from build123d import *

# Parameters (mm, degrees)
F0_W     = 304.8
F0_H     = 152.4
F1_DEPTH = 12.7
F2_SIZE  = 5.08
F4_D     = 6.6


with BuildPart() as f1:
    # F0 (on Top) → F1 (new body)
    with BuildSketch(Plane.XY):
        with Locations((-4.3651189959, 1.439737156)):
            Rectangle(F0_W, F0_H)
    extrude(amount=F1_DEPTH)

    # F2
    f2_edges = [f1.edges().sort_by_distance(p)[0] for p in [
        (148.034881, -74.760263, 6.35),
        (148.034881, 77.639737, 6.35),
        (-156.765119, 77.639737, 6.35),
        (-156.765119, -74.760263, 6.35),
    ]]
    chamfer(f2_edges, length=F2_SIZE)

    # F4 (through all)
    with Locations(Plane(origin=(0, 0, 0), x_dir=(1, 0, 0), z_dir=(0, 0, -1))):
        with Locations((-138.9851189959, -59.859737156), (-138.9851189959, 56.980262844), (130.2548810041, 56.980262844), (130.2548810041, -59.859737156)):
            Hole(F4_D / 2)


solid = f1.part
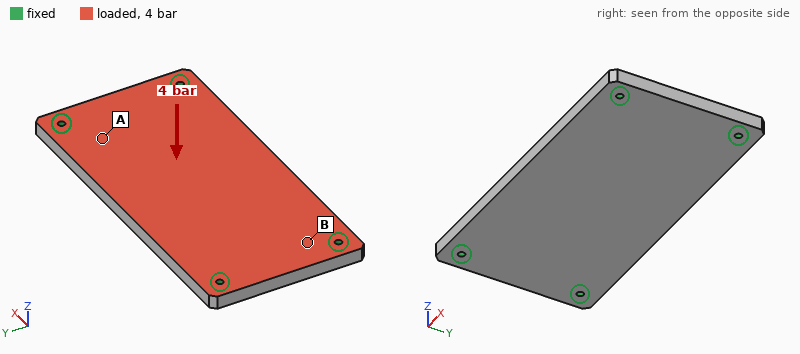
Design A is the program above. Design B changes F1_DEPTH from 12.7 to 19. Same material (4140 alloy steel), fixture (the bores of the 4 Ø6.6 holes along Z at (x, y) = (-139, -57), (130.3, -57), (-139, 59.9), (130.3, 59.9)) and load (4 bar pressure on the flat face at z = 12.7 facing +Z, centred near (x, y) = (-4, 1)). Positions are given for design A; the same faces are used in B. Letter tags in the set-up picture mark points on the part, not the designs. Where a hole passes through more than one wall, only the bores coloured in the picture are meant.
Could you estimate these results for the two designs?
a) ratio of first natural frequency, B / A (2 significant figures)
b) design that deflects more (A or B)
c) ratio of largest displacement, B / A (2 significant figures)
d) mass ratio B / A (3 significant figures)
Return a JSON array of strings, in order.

["1.4", "A", "0.33", "1.50"]
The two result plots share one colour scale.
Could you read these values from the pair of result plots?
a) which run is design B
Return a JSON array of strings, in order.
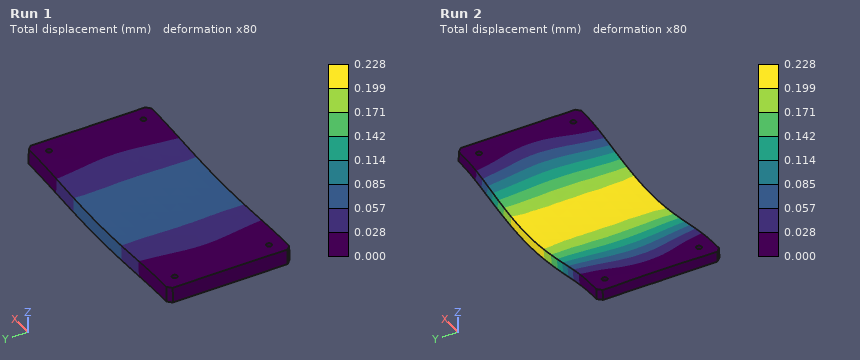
["Run 1"]
